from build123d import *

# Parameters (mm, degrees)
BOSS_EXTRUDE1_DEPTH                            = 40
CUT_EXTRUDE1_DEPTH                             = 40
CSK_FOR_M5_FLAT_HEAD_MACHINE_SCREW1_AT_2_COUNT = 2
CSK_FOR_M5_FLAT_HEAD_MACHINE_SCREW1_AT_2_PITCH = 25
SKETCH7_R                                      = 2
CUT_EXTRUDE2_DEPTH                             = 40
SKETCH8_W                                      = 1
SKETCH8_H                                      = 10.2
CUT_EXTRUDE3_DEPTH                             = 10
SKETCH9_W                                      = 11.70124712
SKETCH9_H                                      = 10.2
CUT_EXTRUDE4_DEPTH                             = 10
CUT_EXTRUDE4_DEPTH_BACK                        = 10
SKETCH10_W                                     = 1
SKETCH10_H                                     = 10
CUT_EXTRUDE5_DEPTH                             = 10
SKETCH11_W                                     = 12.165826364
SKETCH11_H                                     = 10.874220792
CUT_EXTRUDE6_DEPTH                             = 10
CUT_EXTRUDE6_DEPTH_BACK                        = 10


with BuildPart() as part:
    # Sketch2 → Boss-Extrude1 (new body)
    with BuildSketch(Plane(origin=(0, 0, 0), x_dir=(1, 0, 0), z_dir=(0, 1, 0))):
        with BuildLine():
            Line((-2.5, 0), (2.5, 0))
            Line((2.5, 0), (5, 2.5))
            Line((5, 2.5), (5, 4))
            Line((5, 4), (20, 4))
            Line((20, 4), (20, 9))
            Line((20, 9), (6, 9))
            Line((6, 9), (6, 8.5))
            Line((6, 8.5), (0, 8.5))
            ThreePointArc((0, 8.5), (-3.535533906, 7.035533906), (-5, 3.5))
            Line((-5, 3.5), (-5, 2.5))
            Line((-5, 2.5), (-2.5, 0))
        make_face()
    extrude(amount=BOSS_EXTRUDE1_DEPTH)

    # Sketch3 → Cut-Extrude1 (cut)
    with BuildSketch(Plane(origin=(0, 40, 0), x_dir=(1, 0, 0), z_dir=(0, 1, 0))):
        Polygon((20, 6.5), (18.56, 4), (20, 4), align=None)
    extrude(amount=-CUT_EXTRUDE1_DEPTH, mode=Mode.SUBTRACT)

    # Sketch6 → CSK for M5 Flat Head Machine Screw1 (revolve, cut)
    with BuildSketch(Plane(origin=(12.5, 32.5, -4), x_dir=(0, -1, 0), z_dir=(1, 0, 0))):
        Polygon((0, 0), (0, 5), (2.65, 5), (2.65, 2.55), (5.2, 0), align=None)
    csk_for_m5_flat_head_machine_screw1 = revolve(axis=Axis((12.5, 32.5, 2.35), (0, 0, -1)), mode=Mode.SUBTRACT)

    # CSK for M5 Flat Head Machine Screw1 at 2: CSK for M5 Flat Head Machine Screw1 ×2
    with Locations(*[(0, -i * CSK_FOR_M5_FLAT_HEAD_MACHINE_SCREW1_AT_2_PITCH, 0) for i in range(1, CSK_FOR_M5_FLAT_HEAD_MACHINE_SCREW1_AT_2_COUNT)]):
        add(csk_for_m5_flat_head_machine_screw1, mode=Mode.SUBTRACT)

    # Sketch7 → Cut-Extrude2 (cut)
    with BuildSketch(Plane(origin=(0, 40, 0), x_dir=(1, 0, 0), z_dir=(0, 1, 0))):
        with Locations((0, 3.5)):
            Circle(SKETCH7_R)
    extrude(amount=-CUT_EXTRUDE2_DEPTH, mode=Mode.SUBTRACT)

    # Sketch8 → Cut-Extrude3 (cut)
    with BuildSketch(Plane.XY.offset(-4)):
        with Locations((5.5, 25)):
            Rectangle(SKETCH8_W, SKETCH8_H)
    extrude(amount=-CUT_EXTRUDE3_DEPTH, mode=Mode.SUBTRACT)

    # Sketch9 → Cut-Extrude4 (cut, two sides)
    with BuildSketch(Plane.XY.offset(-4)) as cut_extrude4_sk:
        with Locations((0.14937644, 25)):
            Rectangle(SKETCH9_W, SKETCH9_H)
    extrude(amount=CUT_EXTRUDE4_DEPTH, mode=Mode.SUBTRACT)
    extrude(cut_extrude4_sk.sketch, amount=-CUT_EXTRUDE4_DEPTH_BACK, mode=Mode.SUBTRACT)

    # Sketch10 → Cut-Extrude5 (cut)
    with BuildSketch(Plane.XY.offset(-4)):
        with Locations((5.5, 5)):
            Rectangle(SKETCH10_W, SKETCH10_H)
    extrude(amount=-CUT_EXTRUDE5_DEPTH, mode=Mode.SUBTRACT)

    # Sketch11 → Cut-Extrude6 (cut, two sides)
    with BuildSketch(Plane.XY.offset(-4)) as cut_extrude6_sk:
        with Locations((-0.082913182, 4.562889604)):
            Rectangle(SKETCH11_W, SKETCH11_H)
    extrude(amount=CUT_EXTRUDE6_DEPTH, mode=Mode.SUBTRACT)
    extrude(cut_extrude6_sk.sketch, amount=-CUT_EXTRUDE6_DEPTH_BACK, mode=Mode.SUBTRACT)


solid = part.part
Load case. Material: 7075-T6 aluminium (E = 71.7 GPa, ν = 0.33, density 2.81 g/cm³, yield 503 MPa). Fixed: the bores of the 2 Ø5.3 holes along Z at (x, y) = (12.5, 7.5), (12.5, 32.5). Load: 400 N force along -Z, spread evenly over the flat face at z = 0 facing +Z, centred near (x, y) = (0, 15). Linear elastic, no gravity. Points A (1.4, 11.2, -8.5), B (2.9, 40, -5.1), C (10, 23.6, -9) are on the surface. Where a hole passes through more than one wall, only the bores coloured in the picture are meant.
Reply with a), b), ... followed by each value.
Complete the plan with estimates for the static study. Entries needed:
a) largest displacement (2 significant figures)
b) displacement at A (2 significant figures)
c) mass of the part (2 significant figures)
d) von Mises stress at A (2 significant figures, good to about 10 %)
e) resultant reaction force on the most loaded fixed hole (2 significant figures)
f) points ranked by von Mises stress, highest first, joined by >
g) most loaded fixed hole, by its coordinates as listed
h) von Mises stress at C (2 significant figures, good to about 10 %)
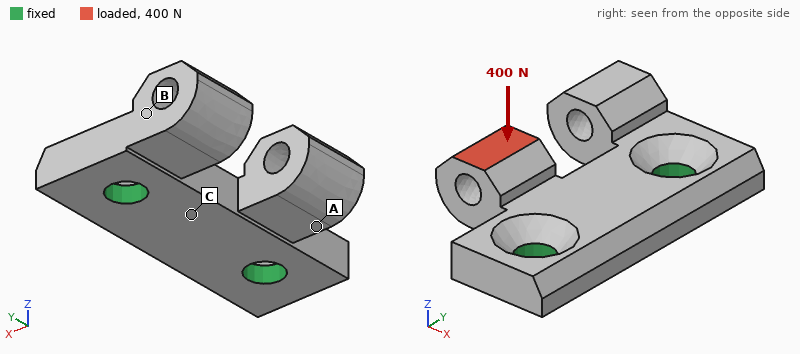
a) 81 µm
b) 39 µm
c) 10 g
d) 24 MPa
e) 340 N
f) C > A > B
g) (12.5, 7.5)
h) 35 MPa
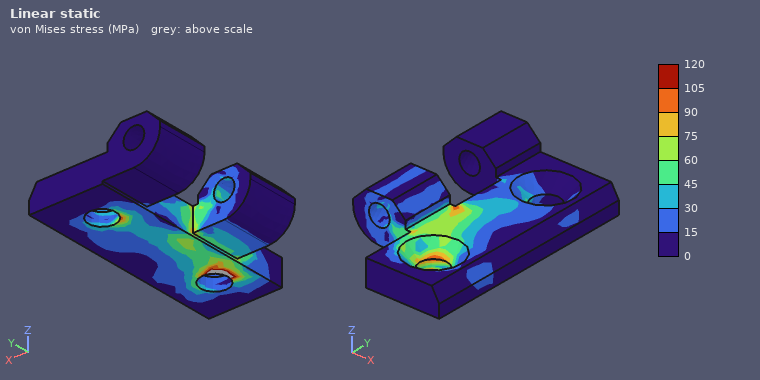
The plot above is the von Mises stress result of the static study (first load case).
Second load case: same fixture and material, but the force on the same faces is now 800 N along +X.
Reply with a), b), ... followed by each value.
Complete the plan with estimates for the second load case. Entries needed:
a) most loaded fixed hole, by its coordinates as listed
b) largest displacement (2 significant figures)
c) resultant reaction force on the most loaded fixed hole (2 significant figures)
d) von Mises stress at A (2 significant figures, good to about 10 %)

a) (12.5, 7.5)
b) 0.12 mm
c) 560 N
d) 50 MPa
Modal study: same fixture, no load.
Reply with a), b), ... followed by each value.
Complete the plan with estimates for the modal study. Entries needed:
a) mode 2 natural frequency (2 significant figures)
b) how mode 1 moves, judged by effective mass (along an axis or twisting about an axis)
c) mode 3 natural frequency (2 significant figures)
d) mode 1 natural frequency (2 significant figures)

a) 10 kHz
b) along Z
c) 20 kHz
d) 9700 Hz
